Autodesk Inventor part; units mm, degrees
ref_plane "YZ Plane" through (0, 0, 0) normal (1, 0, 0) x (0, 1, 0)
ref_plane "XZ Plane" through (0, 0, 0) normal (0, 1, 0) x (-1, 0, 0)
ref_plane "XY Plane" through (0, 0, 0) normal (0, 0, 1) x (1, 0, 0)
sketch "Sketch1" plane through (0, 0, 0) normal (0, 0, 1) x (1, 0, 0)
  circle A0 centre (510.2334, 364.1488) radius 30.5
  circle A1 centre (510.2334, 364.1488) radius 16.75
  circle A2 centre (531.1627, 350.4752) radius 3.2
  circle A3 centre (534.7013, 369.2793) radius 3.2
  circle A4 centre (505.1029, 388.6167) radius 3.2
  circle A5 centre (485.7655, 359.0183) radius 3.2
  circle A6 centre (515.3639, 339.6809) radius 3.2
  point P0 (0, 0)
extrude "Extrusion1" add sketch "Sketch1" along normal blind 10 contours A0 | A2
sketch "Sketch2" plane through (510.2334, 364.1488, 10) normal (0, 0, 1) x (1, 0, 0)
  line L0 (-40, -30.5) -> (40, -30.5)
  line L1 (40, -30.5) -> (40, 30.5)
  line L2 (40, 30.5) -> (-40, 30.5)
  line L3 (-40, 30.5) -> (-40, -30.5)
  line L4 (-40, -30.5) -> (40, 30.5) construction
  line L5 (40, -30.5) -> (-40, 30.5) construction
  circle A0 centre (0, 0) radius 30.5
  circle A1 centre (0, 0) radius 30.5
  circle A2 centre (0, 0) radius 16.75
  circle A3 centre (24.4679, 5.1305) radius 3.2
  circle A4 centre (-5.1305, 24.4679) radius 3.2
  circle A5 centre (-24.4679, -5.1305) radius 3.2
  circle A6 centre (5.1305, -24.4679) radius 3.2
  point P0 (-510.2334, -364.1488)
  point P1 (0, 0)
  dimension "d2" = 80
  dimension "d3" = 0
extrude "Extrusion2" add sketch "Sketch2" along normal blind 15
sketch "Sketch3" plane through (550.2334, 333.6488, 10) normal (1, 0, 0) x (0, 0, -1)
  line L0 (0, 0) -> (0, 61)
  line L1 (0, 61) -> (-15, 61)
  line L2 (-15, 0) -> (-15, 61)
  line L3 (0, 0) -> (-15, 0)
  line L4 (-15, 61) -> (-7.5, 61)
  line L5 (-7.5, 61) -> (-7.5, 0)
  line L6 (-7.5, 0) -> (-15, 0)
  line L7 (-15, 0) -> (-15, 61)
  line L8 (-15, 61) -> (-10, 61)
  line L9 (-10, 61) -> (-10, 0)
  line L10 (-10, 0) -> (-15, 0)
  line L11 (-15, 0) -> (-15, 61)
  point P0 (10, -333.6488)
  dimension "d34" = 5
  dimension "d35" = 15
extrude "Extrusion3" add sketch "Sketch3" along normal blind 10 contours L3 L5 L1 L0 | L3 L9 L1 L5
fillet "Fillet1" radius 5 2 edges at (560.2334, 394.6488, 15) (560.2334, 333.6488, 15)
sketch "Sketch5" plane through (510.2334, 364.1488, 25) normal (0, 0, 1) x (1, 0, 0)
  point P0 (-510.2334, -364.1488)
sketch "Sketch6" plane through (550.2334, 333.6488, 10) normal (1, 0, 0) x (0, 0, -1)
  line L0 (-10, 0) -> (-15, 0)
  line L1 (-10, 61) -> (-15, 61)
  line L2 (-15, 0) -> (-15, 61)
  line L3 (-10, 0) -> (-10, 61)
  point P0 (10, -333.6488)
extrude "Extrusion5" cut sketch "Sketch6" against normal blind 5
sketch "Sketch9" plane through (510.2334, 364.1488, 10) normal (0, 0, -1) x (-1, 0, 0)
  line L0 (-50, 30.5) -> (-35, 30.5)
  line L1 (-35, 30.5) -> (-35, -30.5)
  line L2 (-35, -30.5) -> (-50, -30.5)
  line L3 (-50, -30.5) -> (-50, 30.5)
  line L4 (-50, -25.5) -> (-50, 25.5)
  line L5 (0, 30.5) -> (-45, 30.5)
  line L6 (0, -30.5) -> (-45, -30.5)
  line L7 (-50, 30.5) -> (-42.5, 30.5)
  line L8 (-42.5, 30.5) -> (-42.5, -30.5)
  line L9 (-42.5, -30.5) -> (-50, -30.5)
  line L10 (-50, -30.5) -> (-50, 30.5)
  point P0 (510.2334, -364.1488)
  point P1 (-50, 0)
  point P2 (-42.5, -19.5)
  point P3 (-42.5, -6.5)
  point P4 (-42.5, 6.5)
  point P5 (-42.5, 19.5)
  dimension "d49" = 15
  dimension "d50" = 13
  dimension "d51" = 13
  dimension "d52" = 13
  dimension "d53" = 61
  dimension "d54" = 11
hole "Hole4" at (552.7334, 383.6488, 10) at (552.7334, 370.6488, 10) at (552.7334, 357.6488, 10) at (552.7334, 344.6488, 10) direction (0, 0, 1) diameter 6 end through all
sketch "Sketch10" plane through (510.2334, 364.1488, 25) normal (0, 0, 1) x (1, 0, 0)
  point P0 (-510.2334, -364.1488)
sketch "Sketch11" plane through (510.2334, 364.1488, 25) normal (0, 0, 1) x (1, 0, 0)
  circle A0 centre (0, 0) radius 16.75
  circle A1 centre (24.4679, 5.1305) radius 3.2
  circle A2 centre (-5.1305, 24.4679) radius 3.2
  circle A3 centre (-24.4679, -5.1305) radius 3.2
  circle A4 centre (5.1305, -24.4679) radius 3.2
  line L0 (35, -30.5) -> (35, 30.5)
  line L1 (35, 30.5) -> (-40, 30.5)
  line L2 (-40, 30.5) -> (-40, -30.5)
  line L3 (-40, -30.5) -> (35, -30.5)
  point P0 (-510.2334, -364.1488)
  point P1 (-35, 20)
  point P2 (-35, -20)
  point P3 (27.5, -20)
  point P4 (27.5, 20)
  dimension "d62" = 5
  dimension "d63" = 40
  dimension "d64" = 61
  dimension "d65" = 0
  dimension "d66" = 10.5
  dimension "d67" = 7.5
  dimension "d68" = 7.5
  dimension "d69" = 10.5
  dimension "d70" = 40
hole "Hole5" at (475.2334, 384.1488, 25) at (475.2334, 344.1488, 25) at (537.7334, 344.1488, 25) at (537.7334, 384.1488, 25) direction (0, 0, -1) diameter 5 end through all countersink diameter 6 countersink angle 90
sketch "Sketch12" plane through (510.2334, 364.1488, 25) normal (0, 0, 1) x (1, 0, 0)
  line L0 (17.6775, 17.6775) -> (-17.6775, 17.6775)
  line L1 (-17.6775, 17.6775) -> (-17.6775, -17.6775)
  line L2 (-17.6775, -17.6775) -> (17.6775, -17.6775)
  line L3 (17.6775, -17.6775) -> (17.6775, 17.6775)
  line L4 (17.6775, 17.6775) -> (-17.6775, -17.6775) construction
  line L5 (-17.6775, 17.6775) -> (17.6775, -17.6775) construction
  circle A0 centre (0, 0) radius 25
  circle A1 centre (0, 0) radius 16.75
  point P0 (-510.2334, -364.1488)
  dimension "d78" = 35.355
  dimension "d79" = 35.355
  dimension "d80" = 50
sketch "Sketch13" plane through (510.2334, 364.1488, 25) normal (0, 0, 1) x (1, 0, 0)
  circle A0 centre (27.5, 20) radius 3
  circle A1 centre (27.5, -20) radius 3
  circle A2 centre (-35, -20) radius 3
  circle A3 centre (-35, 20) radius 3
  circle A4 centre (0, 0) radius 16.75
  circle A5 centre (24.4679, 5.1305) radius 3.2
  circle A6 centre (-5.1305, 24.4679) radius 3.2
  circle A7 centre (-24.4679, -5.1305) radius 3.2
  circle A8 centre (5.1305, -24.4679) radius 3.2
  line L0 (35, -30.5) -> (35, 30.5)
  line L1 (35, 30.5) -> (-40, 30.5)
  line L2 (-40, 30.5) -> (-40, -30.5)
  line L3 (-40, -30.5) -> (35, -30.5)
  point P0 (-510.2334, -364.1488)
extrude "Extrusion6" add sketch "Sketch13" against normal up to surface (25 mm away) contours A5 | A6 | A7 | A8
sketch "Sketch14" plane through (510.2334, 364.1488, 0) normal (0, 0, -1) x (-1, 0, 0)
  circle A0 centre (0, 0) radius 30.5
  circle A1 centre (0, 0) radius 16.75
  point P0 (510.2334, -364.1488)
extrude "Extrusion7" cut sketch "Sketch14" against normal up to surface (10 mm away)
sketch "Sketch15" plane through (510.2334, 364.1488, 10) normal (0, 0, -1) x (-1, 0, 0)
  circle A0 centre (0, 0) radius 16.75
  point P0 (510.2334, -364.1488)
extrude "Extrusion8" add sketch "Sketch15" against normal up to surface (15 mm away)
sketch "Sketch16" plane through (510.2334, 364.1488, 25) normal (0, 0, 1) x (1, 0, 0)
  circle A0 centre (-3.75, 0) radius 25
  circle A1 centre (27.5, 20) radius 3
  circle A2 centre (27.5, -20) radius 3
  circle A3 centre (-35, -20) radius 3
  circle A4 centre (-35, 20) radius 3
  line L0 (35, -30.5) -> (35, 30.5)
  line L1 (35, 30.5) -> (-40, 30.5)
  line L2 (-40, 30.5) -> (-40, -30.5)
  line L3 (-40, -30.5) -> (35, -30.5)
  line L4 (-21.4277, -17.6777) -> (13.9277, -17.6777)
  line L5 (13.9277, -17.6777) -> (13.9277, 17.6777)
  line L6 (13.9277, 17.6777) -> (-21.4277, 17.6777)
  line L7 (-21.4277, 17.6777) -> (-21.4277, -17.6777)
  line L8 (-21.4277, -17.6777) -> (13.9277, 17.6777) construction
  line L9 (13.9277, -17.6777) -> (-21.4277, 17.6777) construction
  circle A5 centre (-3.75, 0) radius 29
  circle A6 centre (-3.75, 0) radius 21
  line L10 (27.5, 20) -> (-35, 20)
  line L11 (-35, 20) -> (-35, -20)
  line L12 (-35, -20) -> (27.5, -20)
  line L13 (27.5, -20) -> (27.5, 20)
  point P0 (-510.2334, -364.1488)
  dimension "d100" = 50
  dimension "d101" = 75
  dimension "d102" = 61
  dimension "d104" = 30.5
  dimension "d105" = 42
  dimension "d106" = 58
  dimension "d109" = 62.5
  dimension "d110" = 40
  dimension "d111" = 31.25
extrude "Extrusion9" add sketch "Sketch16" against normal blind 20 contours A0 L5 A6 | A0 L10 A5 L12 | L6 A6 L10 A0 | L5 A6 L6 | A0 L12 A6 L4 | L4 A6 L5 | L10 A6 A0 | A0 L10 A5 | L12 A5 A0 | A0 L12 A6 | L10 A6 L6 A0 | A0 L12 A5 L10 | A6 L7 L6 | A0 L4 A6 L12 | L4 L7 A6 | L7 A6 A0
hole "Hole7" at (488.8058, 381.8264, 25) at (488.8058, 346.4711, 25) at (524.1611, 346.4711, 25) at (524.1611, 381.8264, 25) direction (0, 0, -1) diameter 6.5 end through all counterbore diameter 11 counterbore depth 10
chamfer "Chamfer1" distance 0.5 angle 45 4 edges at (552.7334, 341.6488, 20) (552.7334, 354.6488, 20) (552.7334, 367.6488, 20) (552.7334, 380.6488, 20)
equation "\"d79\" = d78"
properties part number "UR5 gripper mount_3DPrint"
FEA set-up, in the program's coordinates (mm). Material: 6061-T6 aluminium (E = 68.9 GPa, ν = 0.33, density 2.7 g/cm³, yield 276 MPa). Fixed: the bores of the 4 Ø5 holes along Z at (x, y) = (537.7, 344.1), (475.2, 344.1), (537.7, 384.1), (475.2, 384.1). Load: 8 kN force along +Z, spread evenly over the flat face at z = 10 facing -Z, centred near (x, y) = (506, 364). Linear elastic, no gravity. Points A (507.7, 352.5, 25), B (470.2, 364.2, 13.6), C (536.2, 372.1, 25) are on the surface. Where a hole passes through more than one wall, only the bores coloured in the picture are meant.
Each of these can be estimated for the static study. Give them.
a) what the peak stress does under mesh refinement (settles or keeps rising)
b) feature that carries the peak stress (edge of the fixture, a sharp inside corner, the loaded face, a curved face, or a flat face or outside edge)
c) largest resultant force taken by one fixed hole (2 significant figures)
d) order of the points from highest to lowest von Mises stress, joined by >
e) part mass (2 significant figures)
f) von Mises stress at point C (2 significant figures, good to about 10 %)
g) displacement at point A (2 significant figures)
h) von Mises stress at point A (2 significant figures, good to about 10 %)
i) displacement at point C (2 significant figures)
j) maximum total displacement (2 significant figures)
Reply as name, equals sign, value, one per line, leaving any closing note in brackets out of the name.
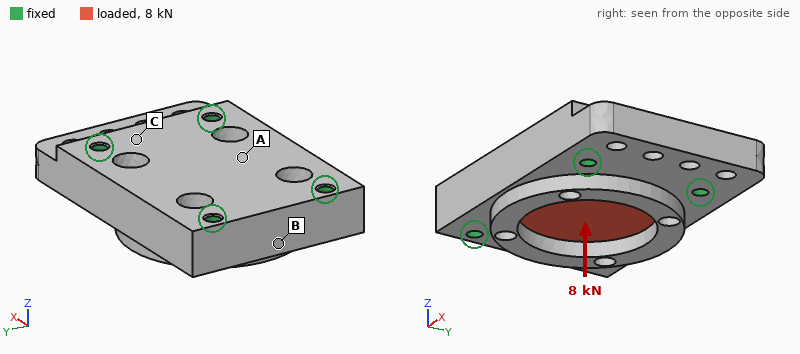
what the peak stress does under mesh refinement = keeps rising
feature that carries the peak stress = edge of the fixture
largest resultant force taken by one fixed hole = 2.0 kN
order of the points from highest to lowest von Mises stress, joined by > = A > C > B
part mass = 210 g
von Mises stress at point C = 8.7 MPa
displacement at point A = 16 µm
von Mises stress at point A = 17 MPa
displacement at point C = 4.9 µm
maximum total displacement = 18 µm
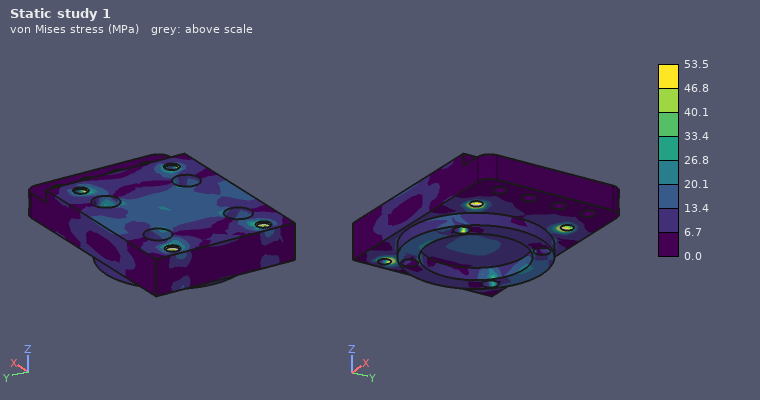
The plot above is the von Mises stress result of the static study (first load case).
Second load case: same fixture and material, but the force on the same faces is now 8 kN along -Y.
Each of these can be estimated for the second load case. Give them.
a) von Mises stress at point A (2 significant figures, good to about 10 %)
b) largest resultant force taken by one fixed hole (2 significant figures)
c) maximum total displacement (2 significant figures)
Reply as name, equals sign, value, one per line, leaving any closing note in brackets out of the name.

von Mises stress at point A = 3.8 MPa
largest resultant force taken by one fixed hole = 2.4 kN
maximum total displacement = 9.1 µm
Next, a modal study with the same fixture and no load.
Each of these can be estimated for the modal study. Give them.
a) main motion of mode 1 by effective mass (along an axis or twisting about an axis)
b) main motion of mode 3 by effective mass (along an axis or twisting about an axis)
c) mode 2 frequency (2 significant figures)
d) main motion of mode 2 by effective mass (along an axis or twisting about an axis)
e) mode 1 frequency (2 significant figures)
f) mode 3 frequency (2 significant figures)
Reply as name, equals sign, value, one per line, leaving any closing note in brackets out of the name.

main motion of mode 1 by effective mass = along Z
main motion of mode 3 by effective mass = along Z
mode 2 frequency = 15 kHz
main motion of mode 2 by effective mass = twisting about X
mode 1 frequency = 12 kHz
mode 3 frequency = 16 kHz
